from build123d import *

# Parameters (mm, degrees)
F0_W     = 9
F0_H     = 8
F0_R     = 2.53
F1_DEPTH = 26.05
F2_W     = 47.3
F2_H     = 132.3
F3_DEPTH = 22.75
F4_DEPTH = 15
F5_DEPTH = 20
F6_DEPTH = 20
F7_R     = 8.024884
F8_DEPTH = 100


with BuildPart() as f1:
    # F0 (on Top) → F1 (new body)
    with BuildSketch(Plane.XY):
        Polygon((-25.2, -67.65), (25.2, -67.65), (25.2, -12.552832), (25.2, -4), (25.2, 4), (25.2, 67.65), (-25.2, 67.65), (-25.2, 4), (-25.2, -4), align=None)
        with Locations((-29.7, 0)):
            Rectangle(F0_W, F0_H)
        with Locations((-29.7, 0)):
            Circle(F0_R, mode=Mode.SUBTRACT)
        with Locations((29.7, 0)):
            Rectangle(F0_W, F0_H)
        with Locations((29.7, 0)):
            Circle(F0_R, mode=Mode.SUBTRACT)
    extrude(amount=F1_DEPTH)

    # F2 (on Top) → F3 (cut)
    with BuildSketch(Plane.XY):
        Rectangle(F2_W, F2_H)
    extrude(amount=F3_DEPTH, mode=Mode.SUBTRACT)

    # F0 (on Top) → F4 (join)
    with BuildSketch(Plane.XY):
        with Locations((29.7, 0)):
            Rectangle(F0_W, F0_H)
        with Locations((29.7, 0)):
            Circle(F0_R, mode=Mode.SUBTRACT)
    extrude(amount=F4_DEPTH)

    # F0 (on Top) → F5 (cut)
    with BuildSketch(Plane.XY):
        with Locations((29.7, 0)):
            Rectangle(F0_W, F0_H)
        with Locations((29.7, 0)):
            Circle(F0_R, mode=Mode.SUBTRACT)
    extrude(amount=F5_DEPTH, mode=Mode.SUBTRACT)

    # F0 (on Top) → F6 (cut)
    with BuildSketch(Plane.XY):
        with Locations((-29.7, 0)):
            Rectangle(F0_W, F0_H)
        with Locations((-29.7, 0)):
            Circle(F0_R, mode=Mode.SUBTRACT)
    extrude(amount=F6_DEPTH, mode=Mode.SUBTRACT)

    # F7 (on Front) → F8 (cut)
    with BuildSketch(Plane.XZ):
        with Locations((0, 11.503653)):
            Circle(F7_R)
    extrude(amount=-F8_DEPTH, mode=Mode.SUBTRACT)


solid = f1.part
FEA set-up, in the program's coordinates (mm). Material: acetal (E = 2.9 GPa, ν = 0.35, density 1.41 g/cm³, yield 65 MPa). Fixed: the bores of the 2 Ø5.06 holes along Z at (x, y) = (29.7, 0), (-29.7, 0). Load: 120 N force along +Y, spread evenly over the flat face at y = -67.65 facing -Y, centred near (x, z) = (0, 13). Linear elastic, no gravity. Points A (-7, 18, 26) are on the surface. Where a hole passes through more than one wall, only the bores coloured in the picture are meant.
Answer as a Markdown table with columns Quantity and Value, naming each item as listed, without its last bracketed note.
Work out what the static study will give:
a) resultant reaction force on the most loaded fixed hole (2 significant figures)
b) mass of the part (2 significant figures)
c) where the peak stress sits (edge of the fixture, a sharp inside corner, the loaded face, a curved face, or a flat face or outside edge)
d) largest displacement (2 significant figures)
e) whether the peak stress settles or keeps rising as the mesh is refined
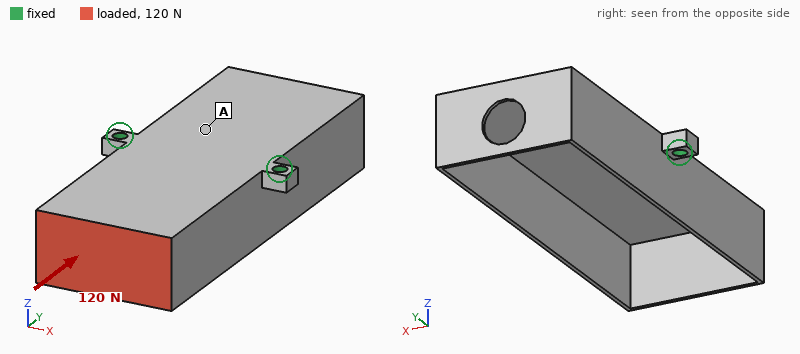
| Quantity | Value |
|---|---|
| resultant reaction force on the most loaded fixed hole | 60 N |
| mass of the part | 50 g |
| where the peak stress sits | edge of the fixture |
| largest displacement | 1.8 mm |
| whether the peak stress settles or keeps rising as the mesh is refined | keeps rising |
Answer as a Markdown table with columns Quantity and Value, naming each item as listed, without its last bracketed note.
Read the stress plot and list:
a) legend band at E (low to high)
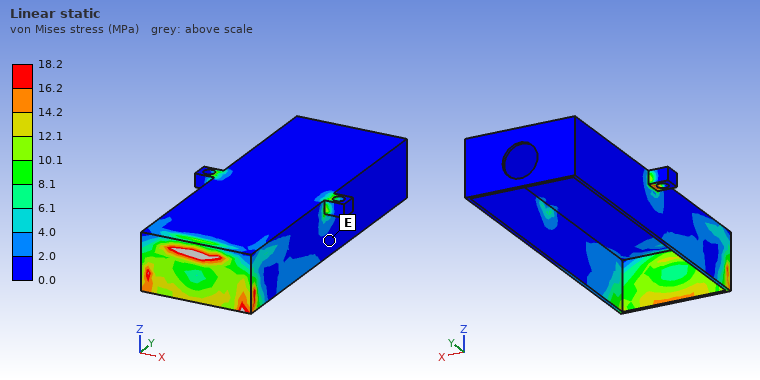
| Quantity | Value |
|---|---|
| legend band at E | 0.0 to 2.0 MPa |
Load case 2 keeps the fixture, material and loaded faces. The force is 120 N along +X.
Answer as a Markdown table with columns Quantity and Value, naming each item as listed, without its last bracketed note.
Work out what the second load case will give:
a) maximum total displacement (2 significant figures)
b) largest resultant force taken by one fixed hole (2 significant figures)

| Quantity | Value |
|---|---|
| maximum total displacement | 1.8 mm |
| largest resultant force taken by one fixed hole | 170 N |
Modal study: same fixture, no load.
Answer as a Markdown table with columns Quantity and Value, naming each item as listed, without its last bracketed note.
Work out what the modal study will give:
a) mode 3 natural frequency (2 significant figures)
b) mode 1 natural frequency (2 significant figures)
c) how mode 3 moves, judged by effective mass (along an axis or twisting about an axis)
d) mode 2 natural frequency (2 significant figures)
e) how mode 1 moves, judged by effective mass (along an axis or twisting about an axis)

| Quantity | Value |
|---|---|
| mode 3 natural frequency | 710 Hz |
| mode 1 natural frequency | 200 Hz |
| how mode 3 moves, judged by effective mass | along Z |
| mode 2 natural frequency | 350 Hz |
| how mode 1 moves, judged by effective mass | twisting about X |
